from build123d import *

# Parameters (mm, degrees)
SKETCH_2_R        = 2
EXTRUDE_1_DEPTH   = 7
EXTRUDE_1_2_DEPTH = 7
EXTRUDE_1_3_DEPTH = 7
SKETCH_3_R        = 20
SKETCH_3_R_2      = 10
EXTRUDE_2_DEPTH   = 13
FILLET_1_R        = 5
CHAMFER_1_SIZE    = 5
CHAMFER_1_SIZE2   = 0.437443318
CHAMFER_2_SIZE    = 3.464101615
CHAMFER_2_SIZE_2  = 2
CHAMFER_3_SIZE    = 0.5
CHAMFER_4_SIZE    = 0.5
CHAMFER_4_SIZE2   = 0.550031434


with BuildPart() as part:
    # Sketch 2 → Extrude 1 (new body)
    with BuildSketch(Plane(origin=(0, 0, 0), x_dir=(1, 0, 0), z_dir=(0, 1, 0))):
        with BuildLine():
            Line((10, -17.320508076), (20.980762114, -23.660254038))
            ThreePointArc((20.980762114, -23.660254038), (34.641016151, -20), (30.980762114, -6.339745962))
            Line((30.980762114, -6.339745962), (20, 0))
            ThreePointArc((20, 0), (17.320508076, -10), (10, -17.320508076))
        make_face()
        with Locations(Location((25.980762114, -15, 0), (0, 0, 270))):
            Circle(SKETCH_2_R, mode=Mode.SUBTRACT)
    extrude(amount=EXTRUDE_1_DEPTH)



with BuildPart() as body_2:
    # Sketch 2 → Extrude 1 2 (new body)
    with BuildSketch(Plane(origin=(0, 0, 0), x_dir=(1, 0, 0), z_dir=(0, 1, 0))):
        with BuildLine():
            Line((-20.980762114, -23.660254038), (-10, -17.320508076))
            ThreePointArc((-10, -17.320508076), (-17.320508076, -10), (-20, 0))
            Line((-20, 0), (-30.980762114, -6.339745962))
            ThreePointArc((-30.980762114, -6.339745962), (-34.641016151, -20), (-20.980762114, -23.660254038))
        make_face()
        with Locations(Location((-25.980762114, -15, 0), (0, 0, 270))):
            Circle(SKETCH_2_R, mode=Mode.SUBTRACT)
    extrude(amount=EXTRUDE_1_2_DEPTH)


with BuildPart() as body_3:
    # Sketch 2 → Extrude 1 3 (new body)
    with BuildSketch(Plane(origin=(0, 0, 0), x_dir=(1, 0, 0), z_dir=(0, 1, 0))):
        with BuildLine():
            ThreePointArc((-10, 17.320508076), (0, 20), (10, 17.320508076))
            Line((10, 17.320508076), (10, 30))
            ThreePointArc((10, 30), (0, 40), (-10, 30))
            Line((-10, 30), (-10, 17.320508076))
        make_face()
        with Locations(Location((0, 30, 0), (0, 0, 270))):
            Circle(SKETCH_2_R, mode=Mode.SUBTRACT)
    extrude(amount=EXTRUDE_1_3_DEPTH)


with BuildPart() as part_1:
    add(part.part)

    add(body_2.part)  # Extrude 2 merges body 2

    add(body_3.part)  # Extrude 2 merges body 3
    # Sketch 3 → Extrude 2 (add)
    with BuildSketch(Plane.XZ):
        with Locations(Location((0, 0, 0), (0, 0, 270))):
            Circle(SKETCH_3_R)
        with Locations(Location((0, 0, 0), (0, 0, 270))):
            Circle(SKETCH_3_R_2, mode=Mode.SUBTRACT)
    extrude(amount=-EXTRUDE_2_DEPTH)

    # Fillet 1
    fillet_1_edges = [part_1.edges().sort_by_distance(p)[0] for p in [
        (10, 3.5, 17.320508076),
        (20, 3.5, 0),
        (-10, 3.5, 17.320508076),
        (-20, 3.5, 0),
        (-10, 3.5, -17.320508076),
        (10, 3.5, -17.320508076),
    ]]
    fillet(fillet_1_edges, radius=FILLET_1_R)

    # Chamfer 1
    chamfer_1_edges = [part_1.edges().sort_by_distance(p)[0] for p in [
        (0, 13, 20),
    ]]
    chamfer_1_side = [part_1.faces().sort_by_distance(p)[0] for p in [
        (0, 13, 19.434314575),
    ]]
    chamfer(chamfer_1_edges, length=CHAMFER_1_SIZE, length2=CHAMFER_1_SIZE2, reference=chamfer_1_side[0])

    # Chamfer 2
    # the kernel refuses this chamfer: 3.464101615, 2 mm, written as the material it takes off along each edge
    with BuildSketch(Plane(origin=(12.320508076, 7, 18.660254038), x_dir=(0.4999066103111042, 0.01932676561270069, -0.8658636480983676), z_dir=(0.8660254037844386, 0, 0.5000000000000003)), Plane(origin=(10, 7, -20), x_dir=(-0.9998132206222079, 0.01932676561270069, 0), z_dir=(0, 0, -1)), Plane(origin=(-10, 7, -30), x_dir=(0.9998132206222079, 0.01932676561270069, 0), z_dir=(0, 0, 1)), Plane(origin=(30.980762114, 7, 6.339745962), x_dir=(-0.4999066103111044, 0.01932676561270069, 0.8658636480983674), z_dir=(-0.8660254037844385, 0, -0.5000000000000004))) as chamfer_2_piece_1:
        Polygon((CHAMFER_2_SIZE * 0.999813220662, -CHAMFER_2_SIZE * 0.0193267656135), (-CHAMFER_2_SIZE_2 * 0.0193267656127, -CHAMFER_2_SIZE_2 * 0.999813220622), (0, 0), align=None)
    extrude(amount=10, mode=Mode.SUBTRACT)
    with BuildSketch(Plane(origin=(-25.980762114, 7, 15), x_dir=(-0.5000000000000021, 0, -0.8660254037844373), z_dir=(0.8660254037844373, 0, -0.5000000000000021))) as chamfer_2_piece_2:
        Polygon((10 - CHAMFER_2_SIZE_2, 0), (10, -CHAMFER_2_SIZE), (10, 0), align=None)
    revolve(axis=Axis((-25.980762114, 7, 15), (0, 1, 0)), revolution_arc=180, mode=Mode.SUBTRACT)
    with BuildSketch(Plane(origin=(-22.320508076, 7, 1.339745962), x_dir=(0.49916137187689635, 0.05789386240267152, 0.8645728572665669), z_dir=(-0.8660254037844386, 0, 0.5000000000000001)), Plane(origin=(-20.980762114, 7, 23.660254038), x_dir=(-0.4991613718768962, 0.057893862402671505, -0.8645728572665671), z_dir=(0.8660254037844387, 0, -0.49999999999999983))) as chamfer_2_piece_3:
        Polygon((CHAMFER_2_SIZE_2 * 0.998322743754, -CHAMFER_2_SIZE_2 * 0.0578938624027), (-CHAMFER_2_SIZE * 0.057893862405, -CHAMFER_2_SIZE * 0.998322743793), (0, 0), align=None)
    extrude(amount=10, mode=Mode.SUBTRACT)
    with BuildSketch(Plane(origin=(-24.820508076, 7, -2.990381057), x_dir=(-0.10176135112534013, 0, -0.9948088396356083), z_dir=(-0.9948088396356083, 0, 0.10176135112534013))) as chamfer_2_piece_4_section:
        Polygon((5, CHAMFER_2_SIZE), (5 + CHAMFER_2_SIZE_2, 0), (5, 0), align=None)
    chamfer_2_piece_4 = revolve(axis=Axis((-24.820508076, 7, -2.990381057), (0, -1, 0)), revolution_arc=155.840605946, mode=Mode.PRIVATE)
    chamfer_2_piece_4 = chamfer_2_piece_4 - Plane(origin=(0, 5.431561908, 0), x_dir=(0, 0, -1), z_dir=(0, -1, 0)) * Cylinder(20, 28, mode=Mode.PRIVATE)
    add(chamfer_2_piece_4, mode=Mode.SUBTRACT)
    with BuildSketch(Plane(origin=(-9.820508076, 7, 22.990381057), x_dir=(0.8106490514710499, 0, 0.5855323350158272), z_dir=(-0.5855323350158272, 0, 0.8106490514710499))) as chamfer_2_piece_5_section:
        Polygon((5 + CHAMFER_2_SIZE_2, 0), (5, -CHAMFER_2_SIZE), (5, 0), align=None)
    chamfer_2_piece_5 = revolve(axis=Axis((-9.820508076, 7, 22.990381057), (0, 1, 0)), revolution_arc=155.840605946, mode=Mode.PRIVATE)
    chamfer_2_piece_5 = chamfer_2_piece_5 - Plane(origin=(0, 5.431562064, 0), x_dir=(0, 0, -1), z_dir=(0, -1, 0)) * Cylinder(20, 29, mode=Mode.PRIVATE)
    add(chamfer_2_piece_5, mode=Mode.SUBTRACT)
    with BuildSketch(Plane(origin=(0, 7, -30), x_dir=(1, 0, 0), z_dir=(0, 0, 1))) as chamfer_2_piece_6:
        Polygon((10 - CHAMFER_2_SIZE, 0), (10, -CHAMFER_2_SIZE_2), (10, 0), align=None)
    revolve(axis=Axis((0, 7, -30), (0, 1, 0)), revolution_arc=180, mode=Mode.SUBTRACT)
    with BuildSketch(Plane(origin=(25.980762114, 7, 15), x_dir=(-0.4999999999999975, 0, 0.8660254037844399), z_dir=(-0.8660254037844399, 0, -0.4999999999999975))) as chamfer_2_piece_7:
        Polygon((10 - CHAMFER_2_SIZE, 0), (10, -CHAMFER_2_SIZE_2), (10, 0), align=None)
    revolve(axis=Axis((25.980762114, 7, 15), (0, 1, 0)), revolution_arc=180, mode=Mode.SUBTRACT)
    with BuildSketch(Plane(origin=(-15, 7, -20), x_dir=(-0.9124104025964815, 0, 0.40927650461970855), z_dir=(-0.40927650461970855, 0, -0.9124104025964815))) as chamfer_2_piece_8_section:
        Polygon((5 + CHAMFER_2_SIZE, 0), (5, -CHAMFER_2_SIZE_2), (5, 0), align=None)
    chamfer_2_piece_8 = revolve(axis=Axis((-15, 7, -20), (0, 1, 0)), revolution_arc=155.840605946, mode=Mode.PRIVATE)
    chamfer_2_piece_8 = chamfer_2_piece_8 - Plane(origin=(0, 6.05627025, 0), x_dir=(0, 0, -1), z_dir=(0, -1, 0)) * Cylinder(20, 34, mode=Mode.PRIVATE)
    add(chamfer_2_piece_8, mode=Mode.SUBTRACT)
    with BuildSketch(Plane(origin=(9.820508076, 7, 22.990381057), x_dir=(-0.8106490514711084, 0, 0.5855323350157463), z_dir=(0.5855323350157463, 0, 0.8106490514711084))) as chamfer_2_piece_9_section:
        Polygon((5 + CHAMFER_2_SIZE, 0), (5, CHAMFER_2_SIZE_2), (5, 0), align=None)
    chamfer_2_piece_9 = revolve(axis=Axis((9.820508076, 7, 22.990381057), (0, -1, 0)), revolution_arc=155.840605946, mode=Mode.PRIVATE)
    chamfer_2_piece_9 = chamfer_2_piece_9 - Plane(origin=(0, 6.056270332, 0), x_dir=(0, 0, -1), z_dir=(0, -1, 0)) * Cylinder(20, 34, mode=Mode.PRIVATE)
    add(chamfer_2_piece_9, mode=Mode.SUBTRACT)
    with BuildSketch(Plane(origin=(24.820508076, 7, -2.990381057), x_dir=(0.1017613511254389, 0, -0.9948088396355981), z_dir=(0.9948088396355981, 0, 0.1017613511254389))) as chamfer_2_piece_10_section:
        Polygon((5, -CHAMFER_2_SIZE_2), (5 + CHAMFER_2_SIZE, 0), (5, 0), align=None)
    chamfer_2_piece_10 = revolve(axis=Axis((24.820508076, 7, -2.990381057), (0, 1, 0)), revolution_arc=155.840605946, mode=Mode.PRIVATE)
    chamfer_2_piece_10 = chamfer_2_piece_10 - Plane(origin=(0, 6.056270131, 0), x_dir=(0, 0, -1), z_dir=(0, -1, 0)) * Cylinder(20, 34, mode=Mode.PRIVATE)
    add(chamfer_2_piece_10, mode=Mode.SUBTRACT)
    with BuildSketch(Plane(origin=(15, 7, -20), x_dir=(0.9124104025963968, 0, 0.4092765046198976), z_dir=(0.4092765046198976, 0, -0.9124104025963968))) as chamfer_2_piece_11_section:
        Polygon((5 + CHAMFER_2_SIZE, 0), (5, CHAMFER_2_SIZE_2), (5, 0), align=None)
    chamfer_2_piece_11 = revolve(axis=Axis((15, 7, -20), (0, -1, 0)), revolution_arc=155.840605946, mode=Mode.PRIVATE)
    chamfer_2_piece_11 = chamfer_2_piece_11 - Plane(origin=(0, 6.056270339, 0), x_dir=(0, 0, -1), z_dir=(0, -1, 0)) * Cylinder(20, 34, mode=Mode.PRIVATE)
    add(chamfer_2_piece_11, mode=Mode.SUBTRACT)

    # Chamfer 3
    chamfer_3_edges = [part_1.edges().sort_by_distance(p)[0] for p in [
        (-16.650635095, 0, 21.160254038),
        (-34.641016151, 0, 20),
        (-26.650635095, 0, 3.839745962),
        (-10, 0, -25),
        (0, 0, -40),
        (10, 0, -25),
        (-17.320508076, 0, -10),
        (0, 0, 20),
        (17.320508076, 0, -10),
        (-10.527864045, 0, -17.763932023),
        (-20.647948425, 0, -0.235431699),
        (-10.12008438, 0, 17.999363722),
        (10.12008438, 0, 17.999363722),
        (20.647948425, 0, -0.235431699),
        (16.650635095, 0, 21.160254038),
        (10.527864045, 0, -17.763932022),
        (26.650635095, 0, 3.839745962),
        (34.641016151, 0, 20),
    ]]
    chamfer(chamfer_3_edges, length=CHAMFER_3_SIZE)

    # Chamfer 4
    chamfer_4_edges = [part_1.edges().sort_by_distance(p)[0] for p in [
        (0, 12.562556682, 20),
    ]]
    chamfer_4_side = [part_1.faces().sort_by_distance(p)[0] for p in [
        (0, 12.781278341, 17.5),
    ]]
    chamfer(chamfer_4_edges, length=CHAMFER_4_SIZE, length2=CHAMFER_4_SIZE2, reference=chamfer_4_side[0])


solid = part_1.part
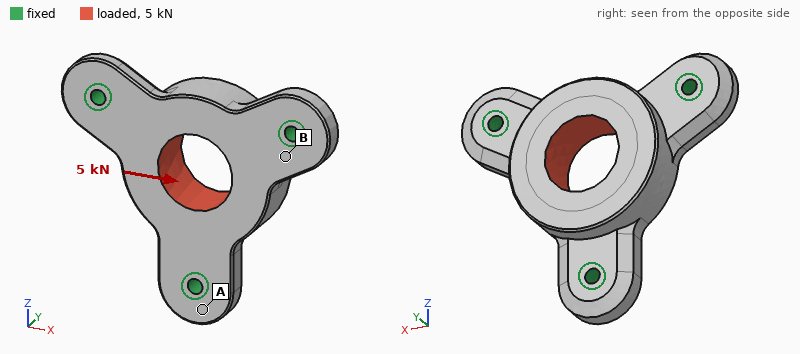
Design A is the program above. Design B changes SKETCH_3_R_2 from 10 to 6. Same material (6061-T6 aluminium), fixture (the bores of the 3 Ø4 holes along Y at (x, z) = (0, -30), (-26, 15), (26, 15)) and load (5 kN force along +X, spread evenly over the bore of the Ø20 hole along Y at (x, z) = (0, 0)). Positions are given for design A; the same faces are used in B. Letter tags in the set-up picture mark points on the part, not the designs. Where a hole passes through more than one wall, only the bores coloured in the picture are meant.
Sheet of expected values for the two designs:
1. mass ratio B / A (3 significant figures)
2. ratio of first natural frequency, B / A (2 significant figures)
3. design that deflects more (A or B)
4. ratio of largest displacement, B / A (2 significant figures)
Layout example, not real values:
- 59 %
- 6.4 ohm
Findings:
- 1.14
- 0.94
- A
- 0.69
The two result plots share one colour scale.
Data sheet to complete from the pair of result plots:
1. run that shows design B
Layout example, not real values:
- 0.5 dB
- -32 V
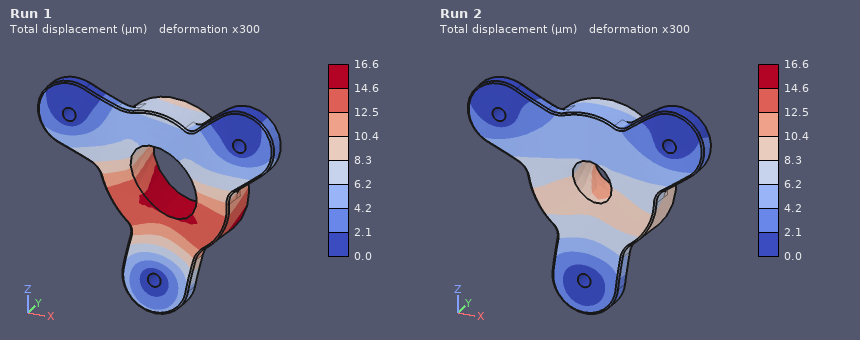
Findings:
- Run 2
